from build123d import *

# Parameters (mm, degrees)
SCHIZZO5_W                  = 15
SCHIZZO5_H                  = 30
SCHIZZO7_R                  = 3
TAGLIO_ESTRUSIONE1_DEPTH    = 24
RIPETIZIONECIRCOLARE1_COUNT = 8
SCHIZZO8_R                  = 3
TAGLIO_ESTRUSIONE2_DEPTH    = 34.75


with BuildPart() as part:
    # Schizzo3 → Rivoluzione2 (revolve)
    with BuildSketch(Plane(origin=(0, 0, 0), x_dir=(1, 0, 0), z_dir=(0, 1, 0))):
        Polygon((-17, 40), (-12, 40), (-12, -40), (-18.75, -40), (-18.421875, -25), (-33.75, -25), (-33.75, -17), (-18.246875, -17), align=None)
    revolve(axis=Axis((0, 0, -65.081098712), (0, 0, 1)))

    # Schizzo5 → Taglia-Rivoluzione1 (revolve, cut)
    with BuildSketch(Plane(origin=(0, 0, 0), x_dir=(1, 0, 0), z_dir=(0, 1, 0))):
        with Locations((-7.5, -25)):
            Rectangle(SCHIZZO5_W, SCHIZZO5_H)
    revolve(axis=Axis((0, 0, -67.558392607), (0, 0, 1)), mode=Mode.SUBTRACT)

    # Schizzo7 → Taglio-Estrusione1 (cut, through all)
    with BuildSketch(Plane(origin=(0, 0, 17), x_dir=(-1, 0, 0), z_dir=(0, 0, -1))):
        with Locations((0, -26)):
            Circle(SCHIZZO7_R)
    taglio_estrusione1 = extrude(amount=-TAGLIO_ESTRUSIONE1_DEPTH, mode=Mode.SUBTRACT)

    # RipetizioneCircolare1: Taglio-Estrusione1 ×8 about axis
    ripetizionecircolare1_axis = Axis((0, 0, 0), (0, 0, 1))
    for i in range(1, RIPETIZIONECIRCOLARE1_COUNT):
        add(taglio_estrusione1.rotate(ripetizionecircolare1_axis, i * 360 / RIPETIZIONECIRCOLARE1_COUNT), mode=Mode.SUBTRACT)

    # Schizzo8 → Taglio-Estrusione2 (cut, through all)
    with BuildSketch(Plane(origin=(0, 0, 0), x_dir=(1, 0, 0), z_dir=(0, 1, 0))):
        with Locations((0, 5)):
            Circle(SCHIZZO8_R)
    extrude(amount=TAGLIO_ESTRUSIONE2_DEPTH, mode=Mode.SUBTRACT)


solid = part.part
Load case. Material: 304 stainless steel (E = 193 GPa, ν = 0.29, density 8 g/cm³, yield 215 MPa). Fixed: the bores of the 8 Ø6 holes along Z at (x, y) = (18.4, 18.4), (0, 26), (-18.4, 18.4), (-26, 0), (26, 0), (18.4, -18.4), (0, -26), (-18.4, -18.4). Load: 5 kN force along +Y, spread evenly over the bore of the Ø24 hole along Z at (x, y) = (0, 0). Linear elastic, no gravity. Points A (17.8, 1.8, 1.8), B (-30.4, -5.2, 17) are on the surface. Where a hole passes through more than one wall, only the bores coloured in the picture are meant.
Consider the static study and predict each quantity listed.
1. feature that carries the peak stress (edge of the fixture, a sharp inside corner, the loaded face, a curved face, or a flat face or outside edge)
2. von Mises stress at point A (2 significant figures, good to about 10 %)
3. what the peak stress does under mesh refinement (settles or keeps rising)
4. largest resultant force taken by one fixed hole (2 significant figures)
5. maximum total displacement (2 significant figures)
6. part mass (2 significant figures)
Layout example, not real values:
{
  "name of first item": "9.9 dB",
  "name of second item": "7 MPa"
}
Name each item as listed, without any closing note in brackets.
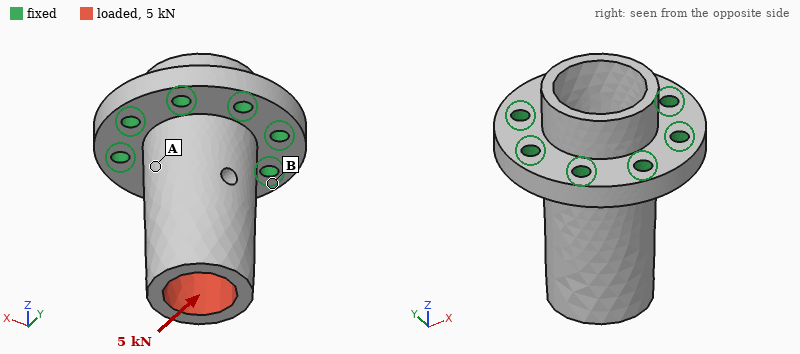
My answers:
{
  "feature that carries the peak stress": "edge of the fixture",
  "von Mises stress at point A": "20 MPa",
  "what the peak stress does under mesh refinement": "keeps rising",
  "largest resultant force taken by one fixed hole": "2.3 kN",
  "maximum total displacement": "32 µm",
  "part mass": "440 g"
}
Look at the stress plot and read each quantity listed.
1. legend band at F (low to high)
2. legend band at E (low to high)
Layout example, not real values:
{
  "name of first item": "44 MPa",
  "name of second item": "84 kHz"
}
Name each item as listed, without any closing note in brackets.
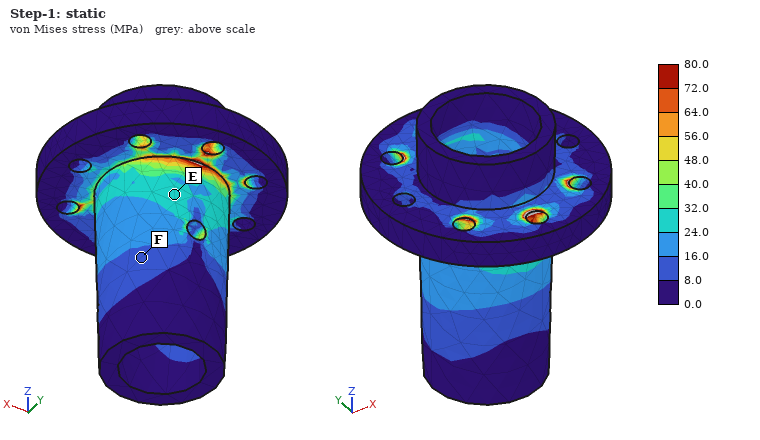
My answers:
{
  "legend band at F": "8.0 to 16.0 MPa",
  "legend band at E": "24.0 to 32.0 MPa"
}
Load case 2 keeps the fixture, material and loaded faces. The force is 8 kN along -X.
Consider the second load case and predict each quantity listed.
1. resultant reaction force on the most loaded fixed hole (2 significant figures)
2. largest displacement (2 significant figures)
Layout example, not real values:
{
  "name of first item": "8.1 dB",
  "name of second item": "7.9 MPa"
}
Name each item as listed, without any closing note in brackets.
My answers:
{
  "resultant reaction force on the most loaded fixed hole": "3.6 kN",
  "largest displacement": "52 µm"
}
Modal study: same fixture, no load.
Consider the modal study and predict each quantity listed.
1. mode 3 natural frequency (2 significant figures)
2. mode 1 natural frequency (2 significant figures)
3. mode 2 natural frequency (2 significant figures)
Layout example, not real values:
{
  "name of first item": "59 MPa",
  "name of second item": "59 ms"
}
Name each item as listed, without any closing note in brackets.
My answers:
{
  "mode 3 natural frequency": "13 kHz",
  "mode 1 natural frequency": "5300 Hz",
  "mode 2 natural frequency": "5300 Hz"
}
